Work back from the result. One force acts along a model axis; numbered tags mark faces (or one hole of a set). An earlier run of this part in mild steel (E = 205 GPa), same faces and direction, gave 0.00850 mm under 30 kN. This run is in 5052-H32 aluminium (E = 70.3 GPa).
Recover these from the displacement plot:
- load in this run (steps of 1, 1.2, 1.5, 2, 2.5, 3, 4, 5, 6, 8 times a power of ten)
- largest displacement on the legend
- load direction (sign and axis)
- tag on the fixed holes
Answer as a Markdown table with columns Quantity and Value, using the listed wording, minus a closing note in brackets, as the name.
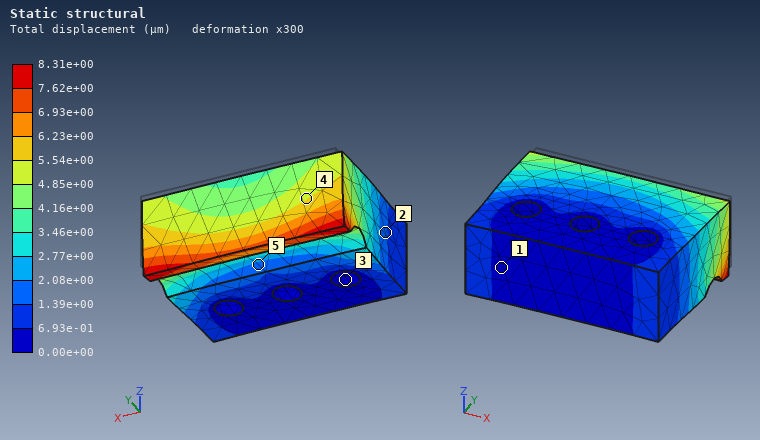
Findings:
| Quantity | Value |
|---|---|
| load in this run | 10 kN |
| largest displacement on the legend | 8.31e+00 µm |
| load direction | -Y |
| tag on the fixed holes | 3 |
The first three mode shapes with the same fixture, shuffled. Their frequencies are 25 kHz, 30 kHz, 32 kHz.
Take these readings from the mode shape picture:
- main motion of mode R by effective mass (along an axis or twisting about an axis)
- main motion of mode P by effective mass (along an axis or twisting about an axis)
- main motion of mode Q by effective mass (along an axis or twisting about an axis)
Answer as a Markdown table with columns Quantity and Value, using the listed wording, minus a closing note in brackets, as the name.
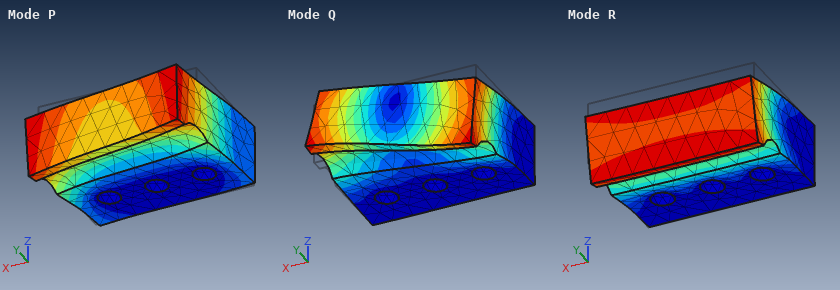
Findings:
| Quantity | Value |
|---|---|
| main motion of mode R by effective mass | along Z |
| main motion of mode P by effective mass | along X |
| main motion of mode Q by effective mass | twisting about Y |
